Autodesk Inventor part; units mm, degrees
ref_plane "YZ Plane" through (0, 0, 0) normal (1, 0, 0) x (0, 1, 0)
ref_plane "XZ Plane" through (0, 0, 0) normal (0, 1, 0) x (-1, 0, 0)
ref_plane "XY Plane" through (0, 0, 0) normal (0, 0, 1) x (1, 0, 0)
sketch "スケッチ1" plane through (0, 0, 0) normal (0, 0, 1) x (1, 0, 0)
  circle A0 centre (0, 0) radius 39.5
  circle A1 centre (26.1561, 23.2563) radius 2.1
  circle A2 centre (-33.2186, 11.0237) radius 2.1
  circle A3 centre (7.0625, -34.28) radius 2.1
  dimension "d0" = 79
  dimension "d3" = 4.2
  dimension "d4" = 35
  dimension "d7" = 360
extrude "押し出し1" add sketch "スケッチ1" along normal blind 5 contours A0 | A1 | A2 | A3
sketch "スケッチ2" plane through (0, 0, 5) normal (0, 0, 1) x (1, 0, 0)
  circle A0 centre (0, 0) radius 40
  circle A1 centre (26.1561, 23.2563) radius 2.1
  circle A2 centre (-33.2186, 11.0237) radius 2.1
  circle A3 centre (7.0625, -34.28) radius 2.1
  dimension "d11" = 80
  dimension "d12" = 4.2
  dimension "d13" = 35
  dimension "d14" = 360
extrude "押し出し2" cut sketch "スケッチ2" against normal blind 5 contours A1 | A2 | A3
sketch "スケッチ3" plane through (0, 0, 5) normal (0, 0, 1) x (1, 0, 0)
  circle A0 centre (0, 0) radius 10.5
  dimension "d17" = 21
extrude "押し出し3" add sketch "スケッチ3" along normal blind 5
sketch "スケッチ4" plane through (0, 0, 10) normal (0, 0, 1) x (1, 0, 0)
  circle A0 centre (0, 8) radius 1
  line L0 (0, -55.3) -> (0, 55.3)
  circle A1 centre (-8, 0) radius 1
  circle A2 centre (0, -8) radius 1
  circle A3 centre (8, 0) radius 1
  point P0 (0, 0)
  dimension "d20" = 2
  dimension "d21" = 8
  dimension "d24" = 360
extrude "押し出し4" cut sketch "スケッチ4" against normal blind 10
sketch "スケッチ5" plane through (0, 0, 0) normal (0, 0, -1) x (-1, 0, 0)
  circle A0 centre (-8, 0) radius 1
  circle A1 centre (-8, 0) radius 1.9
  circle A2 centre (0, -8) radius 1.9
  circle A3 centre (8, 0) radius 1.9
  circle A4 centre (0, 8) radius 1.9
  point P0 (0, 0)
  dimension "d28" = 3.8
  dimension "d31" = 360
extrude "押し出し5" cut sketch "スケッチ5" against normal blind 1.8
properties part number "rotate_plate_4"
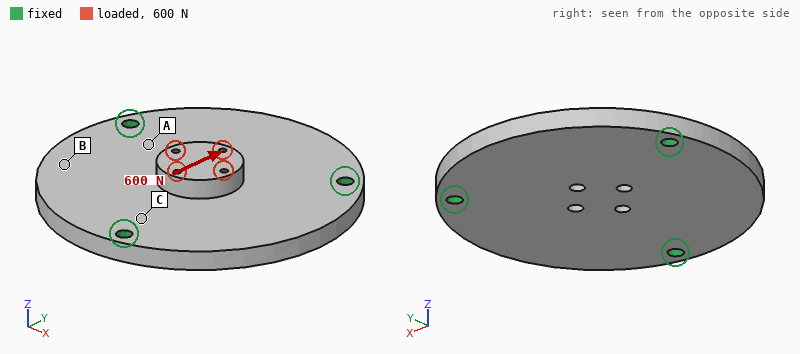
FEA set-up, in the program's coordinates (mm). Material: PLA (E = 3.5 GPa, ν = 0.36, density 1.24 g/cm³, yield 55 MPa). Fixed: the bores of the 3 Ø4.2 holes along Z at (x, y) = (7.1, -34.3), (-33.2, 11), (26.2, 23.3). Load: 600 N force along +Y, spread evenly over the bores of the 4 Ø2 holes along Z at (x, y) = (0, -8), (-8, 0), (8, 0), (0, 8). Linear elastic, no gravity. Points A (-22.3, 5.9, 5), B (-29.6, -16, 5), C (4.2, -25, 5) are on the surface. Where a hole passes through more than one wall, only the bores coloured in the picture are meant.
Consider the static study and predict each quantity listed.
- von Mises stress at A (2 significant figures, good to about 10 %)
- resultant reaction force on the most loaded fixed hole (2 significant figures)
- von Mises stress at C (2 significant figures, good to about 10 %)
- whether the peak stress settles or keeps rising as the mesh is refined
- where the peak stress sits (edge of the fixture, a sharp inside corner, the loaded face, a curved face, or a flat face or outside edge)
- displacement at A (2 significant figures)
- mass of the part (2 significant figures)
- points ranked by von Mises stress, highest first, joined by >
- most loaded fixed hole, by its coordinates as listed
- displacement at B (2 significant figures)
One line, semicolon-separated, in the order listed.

2.3 MPa; 230 N; 3.6 MPa; keeps rising; edge of the fixture; 16 µm; 32 g; C > A > B; (7.1, -34.3); 34 µm
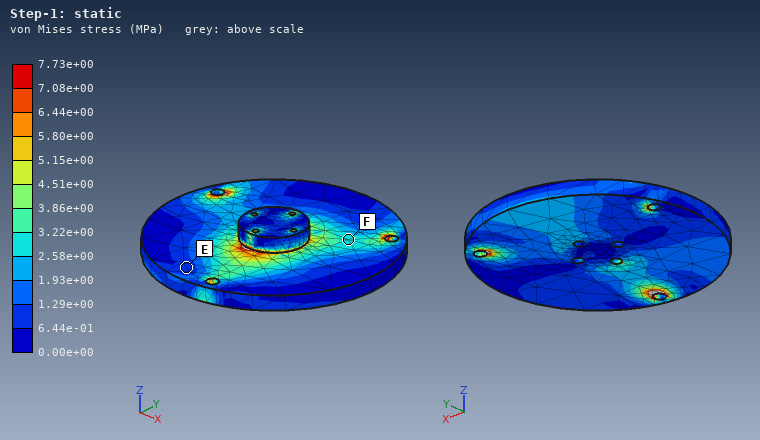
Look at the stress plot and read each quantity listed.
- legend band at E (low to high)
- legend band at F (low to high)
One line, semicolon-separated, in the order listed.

6.44e-01 to 1.29e+00 MPa; 2.58e+00 to 3.22e+00 MPa
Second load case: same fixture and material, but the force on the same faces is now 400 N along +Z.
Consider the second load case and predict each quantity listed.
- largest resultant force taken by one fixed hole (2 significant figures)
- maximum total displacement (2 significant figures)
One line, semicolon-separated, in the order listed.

140 N; 0.24 mm
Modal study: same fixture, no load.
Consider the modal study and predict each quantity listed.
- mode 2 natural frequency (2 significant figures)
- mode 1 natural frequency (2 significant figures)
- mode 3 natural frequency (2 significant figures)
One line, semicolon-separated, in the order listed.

1700 Hz; 1700 Hz; 1700 Hz
